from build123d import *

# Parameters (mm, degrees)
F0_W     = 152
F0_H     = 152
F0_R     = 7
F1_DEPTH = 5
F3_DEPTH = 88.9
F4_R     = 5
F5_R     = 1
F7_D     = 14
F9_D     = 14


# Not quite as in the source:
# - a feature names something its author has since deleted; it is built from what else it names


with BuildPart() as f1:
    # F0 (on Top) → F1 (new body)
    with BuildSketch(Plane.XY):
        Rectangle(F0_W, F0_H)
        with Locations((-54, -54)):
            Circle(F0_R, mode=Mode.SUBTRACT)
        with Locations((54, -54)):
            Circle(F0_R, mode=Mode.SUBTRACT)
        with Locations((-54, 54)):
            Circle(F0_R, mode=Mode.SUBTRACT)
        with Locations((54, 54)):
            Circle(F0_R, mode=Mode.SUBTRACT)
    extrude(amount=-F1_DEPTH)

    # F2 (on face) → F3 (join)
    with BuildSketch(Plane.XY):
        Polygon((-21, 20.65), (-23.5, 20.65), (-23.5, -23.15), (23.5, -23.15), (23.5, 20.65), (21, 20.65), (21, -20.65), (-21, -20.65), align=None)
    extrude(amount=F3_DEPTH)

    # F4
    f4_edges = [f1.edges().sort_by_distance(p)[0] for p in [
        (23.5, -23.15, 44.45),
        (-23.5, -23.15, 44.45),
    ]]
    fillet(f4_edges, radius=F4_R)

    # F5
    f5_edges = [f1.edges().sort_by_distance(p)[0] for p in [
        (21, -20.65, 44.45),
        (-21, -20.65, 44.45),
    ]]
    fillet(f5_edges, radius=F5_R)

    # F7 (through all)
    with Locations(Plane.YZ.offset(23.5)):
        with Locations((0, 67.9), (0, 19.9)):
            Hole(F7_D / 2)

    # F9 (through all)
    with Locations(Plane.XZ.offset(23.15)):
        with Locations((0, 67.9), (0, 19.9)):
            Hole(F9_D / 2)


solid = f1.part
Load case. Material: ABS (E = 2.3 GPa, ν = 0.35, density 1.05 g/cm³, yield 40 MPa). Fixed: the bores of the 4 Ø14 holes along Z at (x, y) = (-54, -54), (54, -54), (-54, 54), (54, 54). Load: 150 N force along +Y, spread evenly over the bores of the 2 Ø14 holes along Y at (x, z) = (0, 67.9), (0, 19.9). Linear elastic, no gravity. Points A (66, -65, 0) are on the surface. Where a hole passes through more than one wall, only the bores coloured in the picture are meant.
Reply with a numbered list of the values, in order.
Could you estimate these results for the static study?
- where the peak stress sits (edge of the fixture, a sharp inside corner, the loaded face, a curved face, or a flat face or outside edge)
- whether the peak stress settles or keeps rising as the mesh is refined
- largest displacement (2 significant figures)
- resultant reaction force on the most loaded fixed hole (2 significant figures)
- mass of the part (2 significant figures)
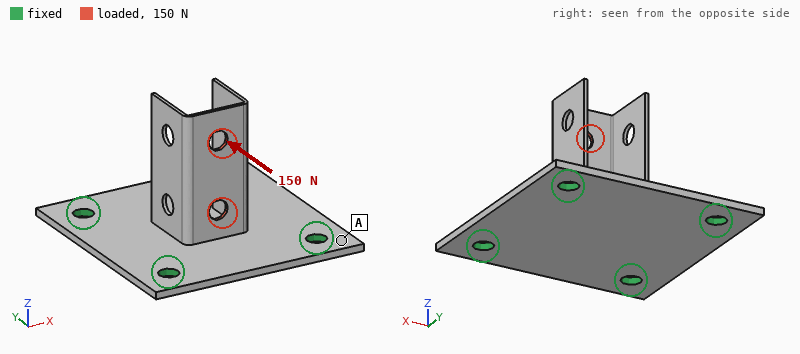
1. a sharp inside corner
2. keeps rising
3. 2.2 mm
4. 59 N
5. 140 g
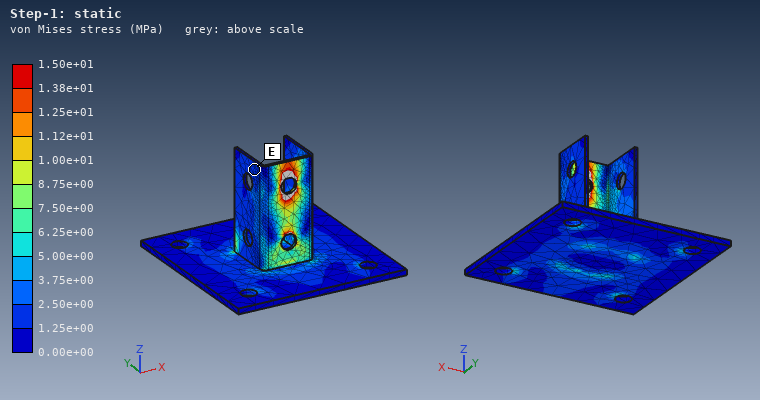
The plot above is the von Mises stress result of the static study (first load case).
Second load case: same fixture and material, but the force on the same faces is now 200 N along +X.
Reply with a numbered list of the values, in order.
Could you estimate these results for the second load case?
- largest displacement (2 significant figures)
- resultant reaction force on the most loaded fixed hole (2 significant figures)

1. 2.5 mm
2. 110 N
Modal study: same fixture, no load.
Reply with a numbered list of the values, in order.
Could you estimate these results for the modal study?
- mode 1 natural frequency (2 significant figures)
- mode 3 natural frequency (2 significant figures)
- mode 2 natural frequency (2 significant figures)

1. 240 Hz
2. 410 Hz
3. 270 Hz
